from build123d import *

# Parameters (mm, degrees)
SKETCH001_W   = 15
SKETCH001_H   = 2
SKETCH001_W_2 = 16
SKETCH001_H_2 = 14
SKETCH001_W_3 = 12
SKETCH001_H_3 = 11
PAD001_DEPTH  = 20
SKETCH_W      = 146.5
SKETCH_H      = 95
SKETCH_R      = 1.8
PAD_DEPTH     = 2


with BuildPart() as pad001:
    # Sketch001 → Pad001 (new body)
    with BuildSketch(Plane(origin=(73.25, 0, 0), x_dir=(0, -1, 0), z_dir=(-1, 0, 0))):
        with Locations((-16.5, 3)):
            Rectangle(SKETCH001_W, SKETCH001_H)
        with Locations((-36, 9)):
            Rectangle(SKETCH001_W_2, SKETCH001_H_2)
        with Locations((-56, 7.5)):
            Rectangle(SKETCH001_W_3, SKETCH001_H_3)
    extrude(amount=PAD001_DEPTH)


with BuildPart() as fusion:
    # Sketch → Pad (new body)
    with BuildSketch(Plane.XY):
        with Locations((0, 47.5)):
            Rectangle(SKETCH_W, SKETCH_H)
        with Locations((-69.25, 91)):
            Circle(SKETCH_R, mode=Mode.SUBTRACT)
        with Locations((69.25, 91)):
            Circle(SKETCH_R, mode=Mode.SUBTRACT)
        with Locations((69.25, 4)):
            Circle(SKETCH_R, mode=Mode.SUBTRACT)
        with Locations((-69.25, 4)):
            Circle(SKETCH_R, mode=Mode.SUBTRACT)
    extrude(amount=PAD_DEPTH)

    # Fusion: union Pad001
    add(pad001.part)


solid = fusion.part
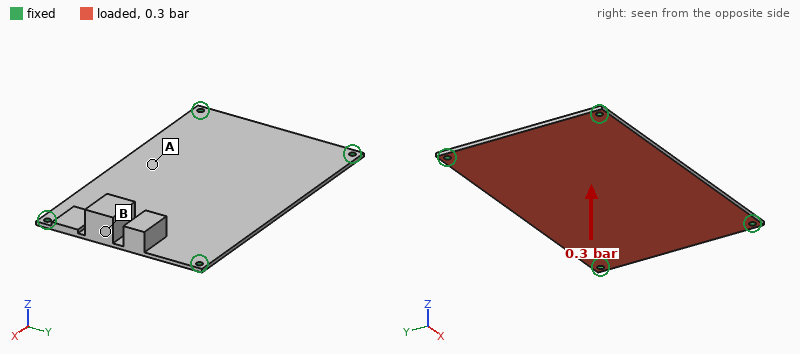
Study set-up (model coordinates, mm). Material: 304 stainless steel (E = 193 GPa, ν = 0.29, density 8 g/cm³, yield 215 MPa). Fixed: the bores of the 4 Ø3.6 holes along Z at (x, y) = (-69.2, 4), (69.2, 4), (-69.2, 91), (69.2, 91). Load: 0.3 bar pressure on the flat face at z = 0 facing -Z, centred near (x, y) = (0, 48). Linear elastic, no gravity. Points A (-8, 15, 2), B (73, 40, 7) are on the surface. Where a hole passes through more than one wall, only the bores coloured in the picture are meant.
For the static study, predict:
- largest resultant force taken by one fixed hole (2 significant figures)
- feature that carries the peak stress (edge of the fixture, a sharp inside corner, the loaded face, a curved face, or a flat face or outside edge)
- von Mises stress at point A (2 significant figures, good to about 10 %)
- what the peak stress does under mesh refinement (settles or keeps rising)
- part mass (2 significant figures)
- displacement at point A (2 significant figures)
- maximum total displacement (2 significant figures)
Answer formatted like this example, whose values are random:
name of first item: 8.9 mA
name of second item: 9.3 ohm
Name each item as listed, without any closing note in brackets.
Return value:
largest resultant force taken by one fixed hole: 120 N
feature that carries the peak stress: edge of the fixture
von Mises stress at point A: 42 MPa
what the peak stress does under mesh refinement: keeps rising
part mass: 280 g
displacement at point A: 0.33 mm
maximum total displacement: 0.35 mm
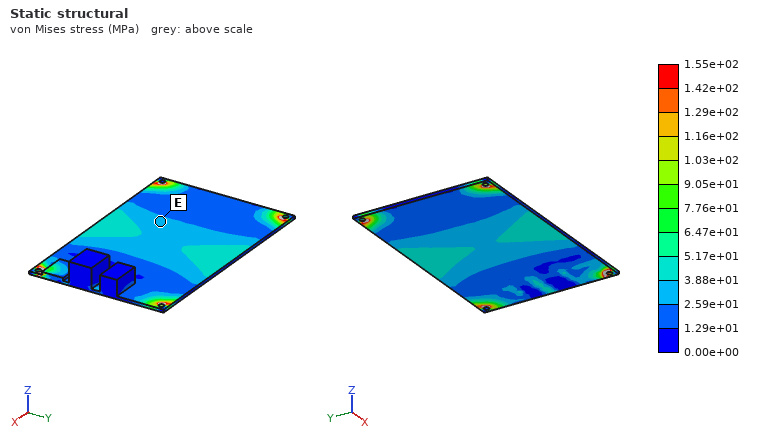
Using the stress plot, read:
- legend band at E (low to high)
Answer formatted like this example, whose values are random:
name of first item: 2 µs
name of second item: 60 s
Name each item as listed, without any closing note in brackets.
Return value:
legend band at E: 2.59e+01 to 3.88e+01 MPa
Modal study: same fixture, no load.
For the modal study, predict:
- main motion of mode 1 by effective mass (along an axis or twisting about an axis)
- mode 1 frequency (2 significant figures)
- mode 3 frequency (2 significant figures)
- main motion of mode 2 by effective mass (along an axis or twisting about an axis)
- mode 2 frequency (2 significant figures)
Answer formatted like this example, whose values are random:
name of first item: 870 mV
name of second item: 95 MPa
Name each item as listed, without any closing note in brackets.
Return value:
main motion of mode 1 by effective mass: along Z
mode 1 frequency: 410 Hz
mode 3 frequency: 860 Hz
main motion of mode 2 by effective mass: twisting about X
mode 2 frequency: 770 Hz
